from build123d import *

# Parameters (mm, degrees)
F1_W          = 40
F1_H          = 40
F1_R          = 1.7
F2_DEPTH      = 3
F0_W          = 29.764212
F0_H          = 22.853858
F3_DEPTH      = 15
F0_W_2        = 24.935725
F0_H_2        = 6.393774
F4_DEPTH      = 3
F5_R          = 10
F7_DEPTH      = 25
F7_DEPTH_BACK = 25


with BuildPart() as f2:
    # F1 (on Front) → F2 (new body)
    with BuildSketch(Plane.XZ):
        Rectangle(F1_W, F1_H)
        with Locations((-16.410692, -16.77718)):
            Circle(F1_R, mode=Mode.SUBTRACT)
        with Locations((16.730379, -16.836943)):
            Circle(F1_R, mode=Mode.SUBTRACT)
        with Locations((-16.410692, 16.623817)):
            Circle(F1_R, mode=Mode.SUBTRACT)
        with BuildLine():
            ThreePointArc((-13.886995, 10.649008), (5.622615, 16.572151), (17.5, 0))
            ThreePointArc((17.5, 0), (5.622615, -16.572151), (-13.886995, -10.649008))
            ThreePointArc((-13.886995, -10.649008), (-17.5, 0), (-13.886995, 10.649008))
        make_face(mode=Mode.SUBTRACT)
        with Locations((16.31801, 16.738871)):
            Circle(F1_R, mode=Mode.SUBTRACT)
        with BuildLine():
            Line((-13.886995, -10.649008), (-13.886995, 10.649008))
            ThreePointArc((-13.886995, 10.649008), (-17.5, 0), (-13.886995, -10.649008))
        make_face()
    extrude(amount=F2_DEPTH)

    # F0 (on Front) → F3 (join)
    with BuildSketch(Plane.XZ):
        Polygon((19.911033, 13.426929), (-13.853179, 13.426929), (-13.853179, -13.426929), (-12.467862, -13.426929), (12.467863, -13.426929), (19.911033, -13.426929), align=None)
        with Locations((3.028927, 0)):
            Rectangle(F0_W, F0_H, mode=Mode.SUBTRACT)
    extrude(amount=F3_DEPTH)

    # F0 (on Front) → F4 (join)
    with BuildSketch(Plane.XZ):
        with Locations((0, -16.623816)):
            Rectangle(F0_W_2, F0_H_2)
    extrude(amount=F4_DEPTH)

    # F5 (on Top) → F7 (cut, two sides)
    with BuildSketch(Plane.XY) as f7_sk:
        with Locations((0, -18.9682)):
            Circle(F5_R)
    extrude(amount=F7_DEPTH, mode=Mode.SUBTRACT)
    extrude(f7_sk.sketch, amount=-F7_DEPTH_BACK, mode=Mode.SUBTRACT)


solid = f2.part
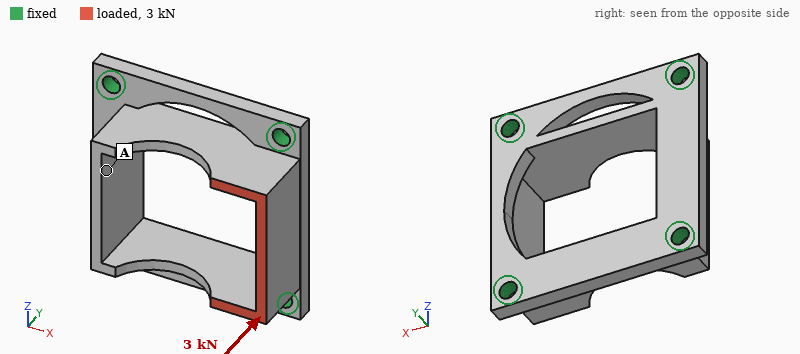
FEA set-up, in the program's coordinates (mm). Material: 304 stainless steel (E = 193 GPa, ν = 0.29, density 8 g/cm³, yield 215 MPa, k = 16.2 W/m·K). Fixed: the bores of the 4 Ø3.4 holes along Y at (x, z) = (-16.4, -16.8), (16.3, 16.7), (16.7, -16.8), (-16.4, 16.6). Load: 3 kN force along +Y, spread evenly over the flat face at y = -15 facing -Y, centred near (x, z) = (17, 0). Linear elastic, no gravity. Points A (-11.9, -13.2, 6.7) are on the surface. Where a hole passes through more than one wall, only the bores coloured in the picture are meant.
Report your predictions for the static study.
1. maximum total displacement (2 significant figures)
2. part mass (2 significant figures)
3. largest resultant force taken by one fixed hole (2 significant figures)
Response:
17 µm
40 g
1.6 kN
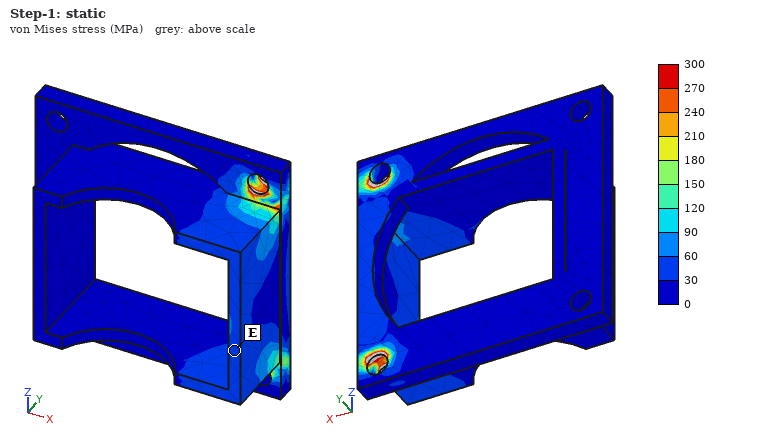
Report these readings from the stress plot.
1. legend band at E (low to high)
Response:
30 to 60 MPa
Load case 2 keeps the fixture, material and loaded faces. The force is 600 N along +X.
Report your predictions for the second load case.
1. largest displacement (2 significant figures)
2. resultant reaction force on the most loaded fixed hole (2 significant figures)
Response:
34 µm
260 N
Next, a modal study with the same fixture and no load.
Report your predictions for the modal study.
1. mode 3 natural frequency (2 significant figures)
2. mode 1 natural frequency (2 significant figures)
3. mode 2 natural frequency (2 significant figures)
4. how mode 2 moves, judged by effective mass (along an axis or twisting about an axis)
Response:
14 kHz
11 kHz
13 kHz
along X
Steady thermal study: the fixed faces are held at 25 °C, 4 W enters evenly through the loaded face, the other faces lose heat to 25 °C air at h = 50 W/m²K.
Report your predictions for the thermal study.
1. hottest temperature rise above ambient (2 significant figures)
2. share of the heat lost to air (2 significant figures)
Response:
40 K
47 %
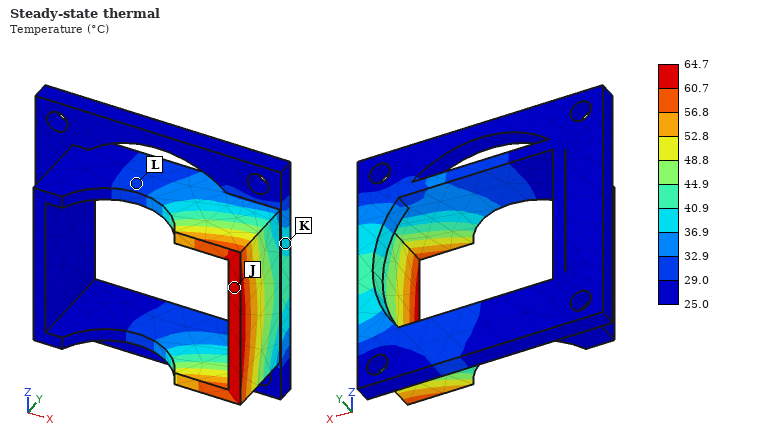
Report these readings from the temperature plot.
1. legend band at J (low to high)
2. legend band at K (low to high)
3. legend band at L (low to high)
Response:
60.7 to 64.7 °C
36.9 to 40.9 °C
29.0 to 32.9 °C
